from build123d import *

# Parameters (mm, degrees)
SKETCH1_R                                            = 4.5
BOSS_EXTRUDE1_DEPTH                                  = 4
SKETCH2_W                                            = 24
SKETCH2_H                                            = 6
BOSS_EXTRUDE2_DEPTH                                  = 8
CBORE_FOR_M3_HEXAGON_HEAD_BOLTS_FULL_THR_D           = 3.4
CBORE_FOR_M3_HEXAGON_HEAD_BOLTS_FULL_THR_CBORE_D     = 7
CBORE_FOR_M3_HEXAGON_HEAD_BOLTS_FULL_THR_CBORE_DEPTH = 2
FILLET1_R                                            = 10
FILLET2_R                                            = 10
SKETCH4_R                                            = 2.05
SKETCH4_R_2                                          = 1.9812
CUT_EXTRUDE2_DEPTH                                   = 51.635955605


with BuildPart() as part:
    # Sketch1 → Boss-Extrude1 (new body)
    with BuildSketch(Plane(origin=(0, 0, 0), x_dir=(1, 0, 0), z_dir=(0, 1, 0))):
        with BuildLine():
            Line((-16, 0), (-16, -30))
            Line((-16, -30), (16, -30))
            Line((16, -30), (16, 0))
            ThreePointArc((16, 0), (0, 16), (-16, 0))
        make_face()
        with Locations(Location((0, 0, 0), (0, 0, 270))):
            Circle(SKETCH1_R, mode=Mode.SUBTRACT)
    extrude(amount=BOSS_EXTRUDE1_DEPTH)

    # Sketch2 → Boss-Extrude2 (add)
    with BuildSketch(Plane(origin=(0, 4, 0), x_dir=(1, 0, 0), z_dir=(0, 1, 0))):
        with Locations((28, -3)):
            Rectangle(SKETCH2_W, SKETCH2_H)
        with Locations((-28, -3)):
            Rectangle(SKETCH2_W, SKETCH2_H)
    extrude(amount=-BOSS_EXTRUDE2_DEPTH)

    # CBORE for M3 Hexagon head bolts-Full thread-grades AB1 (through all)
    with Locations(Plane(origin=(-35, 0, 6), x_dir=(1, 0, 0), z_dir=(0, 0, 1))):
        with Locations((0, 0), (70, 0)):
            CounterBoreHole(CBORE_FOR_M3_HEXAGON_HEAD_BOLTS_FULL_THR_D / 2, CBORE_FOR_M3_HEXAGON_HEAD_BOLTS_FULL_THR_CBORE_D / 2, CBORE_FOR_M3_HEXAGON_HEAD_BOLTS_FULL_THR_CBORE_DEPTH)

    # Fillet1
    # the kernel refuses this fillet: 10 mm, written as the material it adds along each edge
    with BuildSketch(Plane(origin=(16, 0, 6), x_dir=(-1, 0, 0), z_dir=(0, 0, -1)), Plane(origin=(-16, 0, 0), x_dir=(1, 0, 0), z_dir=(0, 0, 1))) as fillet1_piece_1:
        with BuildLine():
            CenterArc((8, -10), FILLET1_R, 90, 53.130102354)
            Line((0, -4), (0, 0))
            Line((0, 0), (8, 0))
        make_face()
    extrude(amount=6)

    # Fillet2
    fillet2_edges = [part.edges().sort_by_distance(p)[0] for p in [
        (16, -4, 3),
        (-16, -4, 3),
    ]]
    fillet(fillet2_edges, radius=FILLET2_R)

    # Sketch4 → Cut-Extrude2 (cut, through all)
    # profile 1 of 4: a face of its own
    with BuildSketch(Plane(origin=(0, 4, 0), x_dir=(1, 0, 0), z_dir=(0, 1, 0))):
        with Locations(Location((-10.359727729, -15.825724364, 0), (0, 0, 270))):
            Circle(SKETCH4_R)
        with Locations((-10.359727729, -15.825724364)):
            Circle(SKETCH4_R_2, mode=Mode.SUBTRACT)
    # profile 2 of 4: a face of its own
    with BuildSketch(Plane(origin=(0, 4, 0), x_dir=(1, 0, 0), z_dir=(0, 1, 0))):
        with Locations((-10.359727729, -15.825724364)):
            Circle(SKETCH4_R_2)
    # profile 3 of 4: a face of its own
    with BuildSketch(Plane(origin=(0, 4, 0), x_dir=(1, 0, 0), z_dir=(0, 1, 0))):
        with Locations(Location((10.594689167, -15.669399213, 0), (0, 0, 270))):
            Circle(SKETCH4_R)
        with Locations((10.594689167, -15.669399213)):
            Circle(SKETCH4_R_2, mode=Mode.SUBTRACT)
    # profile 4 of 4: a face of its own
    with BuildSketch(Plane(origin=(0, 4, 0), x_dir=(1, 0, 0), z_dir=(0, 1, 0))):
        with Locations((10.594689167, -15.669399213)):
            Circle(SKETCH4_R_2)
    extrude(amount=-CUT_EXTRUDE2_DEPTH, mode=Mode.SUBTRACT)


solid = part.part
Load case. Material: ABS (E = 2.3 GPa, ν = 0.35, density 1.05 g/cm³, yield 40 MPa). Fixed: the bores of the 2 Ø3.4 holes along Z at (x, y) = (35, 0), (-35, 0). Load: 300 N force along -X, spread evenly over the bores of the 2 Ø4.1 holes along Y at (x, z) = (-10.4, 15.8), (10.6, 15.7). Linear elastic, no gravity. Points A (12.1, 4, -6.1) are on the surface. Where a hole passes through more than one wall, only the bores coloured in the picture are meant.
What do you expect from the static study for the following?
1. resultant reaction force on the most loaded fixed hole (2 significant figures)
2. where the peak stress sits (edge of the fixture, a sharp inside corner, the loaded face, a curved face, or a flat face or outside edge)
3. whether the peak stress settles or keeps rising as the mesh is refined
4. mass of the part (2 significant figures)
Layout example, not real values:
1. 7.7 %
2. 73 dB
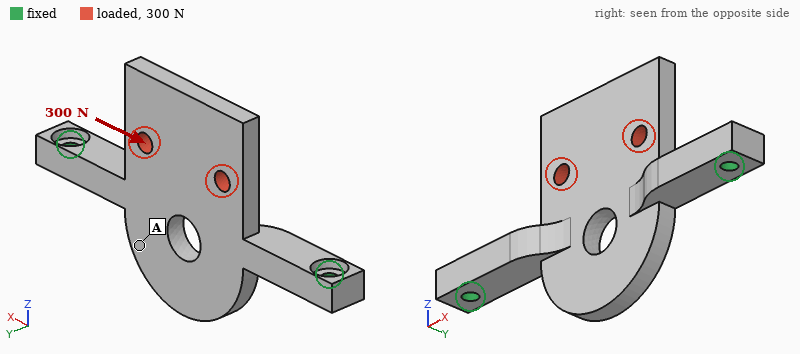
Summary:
1. 170 N
2. edge of the fixture
3. keeps rising
4. 7.6 g
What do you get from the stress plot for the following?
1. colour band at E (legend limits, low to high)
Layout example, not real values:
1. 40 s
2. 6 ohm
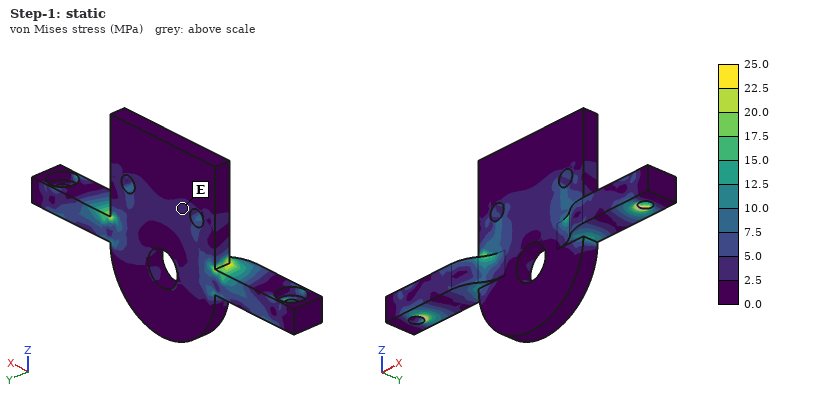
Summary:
1. 2.5 to 5.0 MPa
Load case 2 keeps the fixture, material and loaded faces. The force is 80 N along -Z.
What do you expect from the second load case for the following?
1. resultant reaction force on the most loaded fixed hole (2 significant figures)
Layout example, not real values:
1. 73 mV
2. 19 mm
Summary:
1. 45 N
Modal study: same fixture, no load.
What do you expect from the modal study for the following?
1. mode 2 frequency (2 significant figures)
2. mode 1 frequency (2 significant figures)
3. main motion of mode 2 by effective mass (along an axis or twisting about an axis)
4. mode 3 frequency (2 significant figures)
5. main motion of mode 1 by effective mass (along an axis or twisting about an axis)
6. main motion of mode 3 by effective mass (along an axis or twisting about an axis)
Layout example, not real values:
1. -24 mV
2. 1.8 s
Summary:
1. 1200 Hz
2. 600 Hz
3. along Y
4. 1400 Hz
5. along Y
6. along Z
